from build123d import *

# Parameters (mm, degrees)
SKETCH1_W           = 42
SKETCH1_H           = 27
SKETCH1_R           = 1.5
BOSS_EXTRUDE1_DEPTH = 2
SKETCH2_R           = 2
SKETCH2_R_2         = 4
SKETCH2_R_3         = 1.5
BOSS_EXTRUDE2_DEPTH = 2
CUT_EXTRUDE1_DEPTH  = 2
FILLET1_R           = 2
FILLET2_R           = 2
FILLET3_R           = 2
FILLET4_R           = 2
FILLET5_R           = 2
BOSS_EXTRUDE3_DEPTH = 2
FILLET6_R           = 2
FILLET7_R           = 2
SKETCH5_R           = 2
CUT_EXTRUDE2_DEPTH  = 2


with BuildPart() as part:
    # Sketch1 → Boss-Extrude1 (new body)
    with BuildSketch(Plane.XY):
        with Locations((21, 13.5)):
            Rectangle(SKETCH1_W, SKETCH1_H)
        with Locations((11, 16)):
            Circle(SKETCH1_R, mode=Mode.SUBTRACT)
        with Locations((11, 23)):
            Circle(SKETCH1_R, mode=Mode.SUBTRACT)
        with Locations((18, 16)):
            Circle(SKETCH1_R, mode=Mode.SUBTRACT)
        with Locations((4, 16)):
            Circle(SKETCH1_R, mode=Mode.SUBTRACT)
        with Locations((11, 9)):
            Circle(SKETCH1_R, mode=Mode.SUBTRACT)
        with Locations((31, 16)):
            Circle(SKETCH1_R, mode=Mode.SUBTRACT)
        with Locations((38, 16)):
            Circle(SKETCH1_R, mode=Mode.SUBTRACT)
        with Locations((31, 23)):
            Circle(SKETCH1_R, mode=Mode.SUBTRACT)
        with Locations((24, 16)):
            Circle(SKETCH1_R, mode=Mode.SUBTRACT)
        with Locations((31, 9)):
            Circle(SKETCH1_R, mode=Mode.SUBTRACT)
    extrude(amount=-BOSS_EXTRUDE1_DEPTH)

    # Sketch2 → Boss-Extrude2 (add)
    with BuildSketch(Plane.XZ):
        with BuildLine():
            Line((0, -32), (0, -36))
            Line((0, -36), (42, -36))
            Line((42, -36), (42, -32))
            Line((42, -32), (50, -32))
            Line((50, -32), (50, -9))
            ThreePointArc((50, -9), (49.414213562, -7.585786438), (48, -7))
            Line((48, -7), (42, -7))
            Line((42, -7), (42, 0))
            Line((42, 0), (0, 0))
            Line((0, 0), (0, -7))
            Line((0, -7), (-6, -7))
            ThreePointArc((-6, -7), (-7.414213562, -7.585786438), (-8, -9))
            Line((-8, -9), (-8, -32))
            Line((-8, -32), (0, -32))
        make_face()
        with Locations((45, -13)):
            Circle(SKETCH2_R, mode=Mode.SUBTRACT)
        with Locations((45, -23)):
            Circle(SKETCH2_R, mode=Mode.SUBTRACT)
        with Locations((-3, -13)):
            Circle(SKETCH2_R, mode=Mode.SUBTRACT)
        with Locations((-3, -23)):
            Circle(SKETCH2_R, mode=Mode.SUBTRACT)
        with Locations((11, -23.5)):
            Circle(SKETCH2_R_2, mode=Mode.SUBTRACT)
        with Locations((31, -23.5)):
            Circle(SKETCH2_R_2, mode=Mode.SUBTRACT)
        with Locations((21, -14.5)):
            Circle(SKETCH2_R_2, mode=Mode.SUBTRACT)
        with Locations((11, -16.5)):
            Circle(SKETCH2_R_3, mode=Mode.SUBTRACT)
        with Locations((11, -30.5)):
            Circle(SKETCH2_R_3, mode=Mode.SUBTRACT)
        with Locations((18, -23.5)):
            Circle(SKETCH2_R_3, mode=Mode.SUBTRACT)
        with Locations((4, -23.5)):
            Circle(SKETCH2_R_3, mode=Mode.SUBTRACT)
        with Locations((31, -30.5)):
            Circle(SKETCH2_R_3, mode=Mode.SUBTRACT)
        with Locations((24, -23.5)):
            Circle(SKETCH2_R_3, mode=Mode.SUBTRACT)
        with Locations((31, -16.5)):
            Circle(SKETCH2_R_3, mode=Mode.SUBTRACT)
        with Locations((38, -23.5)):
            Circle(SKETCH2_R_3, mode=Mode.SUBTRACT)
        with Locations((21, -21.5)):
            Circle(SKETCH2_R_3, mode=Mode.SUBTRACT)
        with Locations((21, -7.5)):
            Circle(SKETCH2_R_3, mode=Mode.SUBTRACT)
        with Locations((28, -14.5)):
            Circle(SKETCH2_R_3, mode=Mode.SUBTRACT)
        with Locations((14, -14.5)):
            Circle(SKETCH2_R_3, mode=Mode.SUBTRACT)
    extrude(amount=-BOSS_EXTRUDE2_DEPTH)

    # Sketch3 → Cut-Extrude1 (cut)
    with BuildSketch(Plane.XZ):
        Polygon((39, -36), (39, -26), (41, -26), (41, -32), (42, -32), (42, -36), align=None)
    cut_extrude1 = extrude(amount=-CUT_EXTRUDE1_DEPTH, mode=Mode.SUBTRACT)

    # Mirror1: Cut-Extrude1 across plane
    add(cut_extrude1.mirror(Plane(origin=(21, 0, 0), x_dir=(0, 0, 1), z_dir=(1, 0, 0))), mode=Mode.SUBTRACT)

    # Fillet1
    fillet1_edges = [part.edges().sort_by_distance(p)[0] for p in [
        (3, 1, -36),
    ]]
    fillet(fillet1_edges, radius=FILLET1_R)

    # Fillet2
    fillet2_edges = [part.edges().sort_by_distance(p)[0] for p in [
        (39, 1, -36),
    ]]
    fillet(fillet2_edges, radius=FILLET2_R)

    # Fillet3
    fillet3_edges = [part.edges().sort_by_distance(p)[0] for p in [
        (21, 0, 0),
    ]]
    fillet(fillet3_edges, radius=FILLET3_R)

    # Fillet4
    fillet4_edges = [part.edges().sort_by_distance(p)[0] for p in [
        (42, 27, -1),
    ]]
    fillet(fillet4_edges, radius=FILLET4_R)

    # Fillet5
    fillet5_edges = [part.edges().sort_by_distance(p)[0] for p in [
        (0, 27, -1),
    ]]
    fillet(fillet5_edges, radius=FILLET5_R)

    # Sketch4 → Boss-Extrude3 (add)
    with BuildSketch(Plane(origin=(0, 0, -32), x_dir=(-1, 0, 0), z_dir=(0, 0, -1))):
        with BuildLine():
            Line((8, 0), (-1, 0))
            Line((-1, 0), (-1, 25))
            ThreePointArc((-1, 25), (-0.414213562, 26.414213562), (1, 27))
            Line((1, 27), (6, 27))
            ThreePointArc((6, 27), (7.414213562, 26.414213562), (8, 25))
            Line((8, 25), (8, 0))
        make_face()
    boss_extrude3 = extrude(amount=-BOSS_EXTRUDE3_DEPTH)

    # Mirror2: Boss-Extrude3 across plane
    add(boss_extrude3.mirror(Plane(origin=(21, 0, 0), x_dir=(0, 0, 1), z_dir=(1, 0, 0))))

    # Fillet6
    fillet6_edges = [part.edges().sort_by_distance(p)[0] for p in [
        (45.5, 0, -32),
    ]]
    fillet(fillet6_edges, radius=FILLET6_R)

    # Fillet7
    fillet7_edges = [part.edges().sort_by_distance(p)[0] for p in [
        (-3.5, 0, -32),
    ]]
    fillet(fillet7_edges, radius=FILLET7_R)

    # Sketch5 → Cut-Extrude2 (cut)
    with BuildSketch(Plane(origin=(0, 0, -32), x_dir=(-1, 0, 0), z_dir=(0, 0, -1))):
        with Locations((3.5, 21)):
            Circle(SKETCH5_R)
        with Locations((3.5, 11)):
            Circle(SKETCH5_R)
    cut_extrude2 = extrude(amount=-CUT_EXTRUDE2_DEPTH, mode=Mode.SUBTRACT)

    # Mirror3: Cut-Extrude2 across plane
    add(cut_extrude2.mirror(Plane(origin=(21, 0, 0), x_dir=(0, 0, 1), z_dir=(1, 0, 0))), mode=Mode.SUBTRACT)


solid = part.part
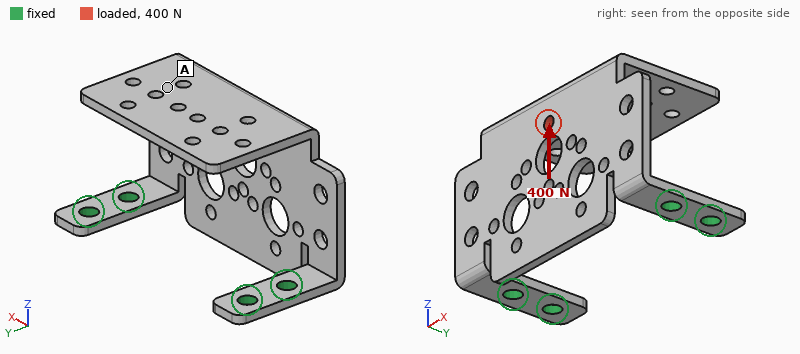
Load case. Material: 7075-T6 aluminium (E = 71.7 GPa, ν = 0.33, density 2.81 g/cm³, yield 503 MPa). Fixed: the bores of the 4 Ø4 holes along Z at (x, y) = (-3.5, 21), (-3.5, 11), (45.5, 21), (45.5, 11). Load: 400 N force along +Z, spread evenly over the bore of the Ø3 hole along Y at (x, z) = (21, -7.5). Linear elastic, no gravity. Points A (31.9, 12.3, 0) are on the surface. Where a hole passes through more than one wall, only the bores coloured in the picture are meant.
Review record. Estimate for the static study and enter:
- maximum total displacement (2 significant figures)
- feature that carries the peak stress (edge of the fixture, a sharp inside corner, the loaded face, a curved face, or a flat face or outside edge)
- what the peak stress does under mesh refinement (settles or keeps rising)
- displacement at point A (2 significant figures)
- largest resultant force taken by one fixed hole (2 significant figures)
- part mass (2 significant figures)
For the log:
0.61 mm
edge of the fixture
keeps rising
0.52 mm
210 N
16 g
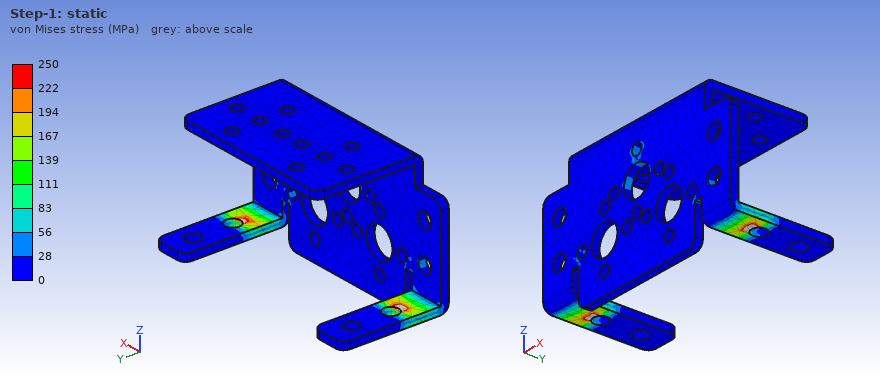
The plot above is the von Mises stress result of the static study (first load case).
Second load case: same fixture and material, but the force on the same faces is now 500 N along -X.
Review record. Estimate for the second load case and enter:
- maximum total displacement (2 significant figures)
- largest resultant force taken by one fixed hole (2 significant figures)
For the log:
0.33 mm
380 N
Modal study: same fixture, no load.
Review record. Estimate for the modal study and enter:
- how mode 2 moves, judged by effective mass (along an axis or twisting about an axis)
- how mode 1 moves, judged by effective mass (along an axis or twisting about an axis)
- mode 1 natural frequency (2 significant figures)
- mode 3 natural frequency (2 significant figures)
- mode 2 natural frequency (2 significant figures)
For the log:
along X
along Y
380 Hz
1400 Hz
1100 Hz
